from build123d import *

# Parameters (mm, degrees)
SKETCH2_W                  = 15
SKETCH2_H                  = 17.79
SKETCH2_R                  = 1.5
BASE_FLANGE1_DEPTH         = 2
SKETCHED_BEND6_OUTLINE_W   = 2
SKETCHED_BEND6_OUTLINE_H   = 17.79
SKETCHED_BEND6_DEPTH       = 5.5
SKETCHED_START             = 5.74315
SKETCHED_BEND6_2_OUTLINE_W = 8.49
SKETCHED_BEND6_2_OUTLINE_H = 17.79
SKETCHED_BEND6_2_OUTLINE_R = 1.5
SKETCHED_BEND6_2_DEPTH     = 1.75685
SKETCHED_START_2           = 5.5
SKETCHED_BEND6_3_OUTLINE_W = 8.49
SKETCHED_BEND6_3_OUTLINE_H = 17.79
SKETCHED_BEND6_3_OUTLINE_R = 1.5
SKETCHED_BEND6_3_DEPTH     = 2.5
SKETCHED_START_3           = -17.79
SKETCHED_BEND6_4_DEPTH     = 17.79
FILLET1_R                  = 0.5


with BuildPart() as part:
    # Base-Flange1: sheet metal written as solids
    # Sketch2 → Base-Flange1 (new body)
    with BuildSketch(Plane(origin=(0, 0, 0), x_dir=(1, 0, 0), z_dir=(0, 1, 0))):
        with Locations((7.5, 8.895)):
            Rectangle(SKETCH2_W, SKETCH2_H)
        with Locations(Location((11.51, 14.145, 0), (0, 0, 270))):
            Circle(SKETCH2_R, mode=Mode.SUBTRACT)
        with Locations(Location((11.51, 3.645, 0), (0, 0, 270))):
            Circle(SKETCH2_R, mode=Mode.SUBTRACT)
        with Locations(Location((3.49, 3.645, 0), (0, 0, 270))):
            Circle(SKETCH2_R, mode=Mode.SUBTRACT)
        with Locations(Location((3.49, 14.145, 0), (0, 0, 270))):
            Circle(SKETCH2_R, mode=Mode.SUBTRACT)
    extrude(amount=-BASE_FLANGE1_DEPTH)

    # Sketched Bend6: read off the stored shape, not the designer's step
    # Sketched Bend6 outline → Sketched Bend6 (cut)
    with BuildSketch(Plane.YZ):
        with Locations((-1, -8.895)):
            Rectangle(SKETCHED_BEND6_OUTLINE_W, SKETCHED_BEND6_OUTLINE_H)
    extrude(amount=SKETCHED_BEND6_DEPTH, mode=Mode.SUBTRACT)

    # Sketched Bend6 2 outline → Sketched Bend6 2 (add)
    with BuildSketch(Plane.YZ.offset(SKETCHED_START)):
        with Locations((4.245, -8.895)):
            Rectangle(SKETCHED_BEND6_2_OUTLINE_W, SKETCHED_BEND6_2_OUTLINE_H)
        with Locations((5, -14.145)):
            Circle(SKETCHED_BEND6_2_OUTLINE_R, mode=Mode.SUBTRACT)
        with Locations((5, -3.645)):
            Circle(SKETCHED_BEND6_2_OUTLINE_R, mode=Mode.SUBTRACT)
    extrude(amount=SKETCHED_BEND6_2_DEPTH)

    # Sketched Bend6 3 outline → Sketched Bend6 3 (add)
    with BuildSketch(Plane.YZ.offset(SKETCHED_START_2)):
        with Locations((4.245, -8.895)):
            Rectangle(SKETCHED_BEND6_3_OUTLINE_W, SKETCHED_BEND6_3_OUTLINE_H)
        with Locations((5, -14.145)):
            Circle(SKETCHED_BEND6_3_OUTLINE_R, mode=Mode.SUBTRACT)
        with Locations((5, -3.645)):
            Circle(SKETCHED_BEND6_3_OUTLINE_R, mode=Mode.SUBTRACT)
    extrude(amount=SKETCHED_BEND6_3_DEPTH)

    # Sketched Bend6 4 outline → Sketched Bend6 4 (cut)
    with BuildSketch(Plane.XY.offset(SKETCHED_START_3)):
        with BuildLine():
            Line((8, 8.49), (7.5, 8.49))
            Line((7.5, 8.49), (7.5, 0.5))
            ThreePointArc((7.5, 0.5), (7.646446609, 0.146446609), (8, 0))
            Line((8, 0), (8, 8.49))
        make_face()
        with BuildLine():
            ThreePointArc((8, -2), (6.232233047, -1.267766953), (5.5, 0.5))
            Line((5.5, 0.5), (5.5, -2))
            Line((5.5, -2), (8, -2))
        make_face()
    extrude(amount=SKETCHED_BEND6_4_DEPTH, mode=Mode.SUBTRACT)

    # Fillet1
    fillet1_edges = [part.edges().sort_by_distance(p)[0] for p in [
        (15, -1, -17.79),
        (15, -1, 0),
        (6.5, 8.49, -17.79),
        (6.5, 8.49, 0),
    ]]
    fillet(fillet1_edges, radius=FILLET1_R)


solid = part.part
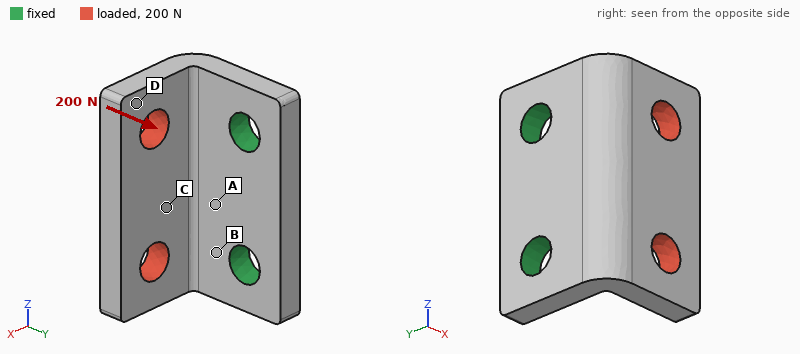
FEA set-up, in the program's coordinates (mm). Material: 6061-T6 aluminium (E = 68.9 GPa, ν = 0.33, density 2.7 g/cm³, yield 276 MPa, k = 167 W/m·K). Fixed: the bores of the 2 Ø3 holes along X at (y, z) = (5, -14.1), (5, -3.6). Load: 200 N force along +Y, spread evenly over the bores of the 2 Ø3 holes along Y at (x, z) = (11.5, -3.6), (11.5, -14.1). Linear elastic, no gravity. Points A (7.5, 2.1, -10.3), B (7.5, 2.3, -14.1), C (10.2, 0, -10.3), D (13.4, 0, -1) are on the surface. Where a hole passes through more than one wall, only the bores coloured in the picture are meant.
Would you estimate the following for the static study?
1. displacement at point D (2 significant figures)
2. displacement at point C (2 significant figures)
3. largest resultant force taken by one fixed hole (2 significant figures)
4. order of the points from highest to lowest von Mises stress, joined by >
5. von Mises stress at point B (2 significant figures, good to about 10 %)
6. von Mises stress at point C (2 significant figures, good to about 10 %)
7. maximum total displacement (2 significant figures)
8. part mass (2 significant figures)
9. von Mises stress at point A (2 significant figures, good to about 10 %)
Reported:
53 µm
27 µm
100 N
B > A > C > D
100 MPa
28 MPa
71 µm
1.5 g
67 MPa
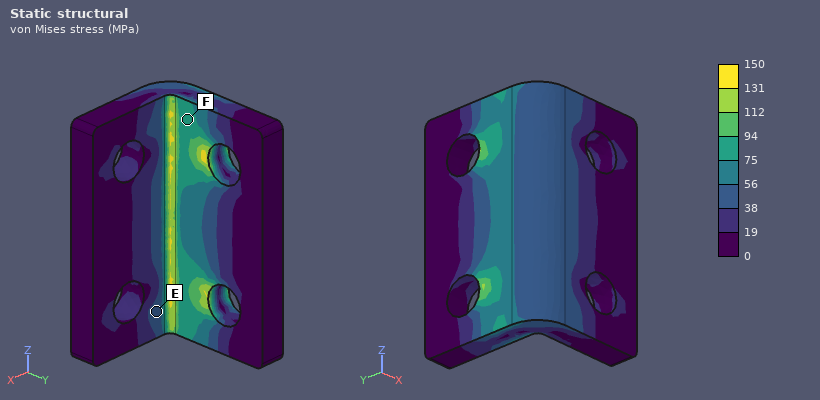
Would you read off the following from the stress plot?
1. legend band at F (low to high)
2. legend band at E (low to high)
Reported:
75 to 94 MPa
38 to 56 MPa
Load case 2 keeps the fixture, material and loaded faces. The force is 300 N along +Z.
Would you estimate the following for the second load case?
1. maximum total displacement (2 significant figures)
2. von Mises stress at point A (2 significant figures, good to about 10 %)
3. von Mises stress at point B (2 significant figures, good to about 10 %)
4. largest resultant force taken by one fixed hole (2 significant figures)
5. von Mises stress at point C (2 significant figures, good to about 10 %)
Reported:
27 µm
44 MPa
57 MPa
230 N
33 MPa
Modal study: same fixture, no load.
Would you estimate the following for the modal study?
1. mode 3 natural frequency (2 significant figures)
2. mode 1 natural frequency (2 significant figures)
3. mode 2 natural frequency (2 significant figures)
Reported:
32 kHz
12 kHz
20 kHz
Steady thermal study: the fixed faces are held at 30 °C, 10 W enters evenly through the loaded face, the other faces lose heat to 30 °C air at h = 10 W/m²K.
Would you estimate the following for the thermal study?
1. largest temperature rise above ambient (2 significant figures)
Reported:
20 K
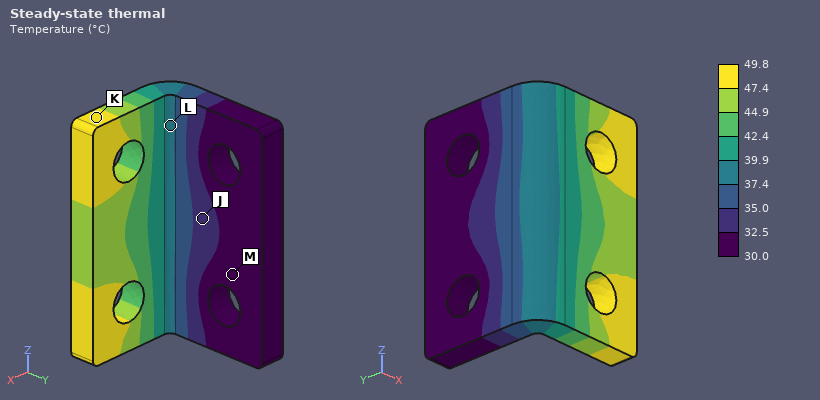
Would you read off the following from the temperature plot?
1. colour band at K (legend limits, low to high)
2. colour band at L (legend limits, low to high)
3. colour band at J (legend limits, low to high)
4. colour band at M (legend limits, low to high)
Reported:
47.4 to 49.8 °C
37.4 to 39.9 °C
32.5 to 35.0 °C
30.0 to 32.5 °C
